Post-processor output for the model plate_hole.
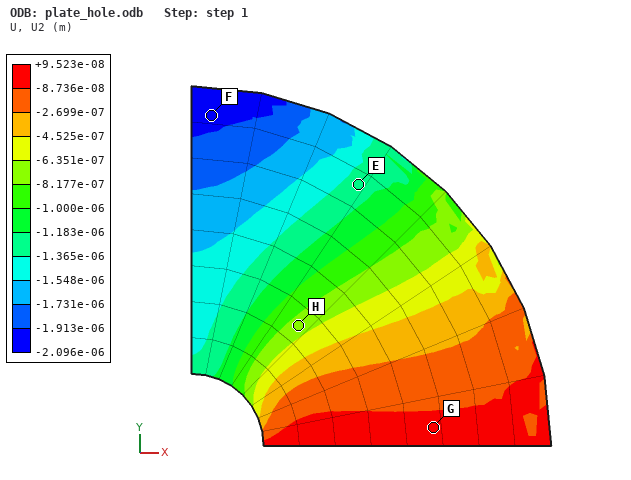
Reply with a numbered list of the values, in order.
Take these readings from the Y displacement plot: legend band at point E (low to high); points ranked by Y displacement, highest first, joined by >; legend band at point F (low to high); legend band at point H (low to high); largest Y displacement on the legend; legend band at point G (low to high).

1. -1.365e-06 to -1.183e-06 m
2. G > H > E > F
3. -2.096e-06 to -1.913e-06 m
4. -8.177e-07 to -6.351e-07 m
5. +9.523e-08 m
6. -8.736e-08 to +9.523e-08 m
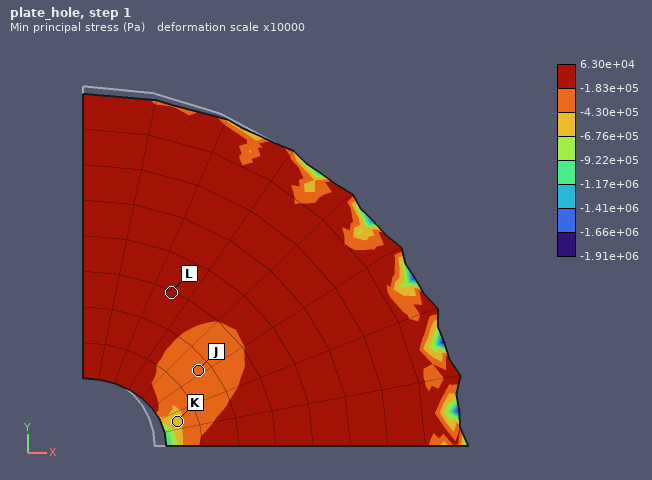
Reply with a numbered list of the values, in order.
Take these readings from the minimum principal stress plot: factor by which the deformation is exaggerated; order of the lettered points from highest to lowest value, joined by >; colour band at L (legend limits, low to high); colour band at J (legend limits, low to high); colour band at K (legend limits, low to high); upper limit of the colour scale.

1. 10000
2. L > J > K
3. -1.83e+05 to 6.30e+04 Pa
4. -4.30e+05 to -1.83e+05 Pa
5. -6.76e+05 to -4.30e+05 Pa
6. 6.30e+04 Pa
